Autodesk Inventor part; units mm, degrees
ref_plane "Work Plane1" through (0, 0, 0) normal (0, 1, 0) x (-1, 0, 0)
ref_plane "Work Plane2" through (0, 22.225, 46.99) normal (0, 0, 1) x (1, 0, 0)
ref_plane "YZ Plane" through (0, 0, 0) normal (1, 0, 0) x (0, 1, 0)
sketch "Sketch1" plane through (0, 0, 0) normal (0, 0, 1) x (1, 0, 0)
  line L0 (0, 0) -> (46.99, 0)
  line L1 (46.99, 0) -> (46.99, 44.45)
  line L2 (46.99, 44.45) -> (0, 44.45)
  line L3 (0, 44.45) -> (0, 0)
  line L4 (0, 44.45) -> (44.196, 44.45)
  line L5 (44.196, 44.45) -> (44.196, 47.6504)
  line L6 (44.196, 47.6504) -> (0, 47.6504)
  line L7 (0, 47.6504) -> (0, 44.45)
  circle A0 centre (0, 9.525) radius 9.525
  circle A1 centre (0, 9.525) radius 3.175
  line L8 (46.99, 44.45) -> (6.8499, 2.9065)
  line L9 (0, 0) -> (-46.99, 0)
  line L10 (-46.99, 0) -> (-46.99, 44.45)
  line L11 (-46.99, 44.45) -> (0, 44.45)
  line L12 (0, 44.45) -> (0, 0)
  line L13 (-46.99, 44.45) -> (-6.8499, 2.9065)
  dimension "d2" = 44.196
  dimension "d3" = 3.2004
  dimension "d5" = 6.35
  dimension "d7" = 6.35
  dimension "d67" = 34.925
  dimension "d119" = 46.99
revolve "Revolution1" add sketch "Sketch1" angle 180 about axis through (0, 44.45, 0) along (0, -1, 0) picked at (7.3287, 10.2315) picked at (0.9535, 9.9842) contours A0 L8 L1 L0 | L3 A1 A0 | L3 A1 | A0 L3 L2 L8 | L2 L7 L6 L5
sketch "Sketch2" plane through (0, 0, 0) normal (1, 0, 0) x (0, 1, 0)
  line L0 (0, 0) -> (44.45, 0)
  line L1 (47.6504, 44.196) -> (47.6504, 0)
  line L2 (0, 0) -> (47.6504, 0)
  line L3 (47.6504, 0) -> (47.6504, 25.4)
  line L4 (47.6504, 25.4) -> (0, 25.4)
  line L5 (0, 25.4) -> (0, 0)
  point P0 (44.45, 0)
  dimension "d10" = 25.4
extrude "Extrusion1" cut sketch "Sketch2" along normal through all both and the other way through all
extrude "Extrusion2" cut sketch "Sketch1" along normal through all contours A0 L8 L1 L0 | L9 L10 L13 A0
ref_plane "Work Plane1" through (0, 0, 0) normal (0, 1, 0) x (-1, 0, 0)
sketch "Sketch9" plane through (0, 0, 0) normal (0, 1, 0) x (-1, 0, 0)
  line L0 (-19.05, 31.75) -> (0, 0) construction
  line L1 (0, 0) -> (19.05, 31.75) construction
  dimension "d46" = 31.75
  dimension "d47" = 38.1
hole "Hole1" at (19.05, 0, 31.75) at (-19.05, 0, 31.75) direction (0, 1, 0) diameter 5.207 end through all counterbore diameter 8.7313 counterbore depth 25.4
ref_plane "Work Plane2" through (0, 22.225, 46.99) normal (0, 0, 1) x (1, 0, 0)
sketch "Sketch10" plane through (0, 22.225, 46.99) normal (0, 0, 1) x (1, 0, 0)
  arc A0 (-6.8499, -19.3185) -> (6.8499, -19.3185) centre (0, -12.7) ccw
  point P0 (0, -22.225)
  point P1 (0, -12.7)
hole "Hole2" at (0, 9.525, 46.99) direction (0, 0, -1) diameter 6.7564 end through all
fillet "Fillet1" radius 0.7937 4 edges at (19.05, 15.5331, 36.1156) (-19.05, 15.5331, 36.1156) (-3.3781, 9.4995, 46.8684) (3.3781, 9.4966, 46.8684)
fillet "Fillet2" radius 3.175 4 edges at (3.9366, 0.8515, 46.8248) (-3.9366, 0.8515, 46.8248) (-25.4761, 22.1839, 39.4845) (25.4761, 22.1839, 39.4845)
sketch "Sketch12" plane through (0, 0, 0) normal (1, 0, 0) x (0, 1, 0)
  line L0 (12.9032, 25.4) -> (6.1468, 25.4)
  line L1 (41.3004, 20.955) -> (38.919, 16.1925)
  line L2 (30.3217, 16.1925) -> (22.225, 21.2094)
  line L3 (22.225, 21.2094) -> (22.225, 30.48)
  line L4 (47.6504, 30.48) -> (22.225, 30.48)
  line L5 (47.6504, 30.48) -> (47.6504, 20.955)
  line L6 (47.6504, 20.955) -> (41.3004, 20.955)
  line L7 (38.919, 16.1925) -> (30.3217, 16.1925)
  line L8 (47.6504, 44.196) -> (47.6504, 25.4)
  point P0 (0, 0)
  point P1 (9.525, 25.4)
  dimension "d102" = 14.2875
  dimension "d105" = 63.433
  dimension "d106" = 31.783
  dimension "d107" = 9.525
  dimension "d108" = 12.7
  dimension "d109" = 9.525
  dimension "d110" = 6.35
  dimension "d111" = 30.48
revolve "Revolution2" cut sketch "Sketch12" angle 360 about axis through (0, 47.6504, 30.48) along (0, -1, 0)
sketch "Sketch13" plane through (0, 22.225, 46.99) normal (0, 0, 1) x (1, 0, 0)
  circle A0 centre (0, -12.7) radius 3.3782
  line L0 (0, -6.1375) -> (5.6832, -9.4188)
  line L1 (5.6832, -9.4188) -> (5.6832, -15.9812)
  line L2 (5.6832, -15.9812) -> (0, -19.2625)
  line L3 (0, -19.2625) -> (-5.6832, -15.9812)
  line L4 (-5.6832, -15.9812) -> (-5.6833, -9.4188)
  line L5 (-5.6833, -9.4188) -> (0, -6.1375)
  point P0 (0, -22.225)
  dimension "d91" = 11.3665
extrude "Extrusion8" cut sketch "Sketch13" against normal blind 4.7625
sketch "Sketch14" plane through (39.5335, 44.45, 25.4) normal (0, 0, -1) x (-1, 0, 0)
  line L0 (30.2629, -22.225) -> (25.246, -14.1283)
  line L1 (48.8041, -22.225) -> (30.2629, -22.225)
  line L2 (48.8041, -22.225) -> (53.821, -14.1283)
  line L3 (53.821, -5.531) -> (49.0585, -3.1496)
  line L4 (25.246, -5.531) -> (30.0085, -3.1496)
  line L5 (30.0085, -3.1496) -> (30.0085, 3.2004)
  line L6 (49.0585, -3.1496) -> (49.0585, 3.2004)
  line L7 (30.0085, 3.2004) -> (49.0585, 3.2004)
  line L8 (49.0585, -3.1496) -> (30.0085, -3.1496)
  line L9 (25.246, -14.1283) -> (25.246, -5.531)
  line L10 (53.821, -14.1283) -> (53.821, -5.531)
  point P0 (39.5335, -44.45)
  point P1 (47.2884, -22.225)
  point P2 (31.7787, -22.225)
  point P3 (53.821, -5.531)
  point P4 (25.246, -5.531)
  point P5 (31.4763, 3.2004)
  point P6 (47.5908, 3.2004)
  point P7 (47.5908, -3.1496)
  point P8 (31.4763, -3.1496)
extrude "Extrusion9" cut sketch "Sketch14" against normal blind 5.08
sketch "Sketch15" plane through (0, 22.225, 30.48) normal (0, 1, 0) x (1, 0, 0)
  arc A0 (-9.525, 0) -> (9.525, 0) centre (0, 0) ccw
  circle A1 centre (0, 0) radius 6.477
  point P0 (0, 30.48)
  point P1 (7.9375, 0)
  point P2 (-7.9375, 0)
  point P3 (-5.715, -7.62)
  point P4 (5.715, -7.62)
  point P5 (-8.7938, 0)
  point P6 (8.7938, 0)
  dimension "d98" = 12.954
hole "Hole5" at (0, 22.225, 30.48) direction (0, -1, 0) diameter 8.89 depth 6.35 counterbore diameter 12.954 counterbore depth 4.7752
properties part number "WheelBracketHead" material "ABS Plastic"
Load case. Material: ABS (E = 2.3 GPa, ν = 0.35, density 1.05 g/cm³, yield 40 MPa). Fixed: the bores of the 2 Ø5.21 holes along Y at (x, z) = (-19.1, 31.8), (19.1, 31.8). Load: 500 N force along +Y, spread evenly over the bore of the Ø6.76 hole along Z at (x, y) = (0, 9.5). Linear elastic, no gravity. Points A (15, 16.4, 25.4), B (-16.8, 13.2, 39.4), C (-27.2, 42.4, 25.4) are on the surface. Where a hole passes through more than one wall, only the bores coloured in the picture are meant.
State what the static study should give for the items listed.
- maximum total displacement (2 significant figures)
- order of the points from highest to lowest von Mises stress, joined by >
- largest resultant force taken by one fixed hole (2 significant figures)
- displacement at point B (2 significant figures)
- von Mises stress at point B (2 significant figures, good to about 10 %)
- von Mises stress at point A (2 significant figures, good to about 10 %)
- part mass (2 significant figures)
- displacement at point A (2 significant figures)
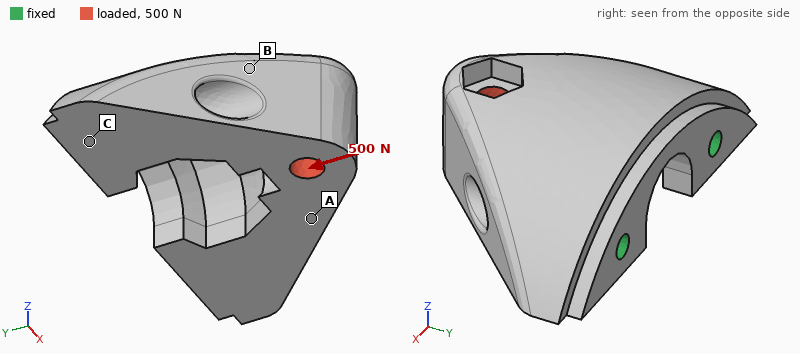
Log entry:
40 µm
A > B > C
280 N
9.2 µm
0.87 MPa
1.9 MPa
30 g
16 µm
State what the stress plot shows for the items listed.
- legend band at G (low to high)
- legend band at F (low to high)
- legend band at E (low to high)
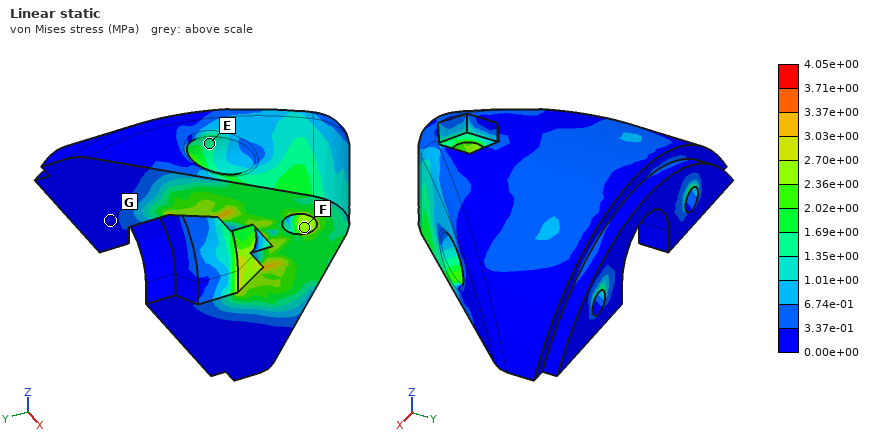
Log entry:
0.00e+00 to 3.37e-01 MPa
2.36e+00 to 2.70e+00 MPa
1.35e+00 to 1.69e+00 MPa
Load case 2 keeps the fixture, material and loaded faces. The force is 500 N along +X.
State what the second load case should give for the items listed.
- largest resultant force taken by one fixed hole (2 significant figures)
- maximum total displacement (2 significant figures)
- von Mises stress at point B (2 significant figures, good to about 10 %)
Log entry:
340 N
62 µm
1.3 MPa
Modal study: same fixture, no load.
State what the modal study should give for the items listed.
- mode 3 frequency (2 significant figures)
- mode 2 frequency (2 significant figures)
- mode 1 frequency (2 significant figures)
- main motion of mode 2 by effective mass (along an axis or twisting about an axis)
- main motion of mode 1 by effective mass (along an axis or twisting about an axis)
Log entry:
7500 Hz
5700 Hz
3100 Hz
along X
along Z
